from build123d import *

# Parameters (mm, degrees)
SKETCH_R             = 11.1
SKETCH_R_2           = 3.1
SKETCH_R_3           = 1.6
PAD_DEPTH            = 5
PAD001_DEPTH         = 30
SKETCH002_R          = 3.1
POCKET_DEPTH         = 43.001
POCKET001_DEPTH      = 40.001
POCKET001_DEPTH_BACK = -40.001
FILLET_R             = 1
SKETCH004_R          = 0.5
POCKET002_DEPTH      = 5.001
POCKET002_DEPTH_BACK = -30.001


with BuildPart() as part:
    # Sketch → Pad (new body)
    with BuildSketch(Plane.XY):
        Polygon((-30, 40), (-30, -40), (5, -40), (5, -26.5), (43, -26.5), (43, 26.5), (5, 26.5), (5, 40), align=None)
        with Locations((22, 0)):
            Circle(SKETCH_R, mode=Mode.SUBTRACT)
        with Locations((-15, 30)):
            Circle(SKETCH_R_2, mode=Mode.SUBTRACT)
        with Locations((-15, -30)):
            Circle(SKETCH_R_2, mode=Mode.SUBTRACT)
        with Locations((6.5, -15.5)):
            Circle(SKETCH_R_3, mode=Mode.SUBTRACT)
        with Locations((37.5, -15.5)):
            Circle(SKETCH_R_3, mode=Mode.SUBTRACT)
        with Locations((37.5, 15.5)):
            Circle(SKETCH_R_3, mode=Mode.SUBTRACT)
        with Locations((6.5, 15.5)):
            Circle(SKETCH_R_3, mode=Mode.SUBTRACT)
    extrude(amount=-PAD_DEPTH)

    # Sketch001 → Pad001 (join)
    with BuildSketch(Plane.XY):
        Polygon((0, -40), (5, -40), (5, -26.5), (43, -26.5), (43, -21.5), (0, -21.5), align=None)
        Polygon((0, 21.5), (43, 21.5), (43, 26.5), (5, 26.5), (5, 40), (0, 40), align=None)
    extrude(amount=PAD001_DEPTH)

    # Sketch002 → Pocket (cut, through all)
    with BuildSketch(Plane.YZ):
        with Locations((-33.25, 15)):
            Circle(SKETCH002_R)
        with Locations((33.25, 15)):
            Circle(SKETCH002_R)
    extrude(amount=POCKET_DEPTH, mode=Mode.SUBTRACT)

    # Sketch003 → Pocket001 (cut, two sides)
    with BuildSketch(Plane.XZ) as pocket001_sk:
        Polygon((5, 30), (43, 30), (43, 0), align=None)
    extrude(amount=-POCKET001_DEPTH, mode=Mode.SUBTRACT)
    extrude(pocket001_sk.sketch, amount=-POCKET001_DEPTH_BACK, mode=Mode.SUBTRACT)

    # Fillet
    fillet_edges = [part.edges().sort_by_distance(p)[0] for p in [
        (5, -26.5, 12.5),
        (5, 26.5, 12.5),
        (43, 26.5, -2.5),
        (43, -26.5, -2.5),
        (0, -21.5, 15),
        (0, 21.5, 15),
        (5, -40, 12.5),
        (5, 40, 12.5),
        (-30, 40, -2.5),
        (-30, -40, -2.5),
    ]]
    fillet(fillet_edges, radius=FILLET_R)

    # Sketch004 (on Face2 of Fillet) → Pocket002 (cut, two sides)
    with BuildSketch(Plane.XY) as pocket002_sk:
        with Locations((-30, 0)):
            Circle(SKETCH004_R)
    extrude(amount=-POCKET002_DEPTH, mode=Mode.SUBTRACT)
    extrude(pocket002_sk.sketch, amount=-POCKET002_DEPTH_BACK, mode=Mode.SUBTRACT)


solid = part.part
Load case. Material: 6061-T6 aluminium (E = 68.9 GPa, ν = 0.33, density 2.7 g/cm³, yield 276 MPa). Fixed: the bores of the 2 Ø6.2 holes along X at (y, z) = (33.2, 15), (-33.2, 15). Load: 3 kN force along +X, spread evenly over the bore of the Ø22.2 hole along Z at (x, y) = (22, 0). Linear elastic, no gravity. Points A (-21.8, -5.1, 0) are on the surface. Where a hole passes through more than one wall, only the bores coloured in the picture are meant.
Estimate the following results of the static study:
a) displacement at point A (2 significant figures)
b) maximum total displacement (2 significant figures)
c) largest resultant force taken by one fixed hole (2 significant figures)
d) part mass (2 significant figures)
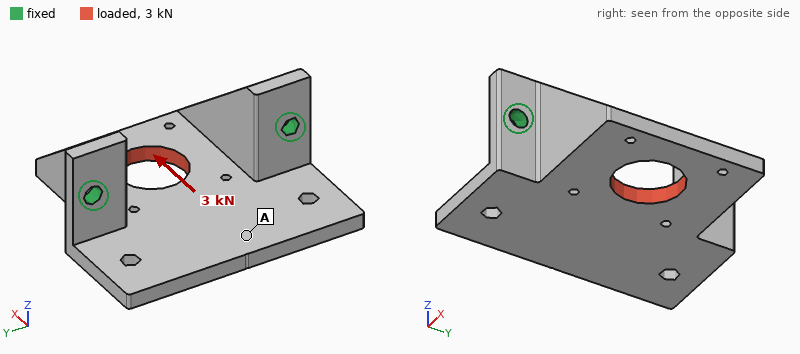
0.16 mm
0.24 mm
1.5 kN
88 g
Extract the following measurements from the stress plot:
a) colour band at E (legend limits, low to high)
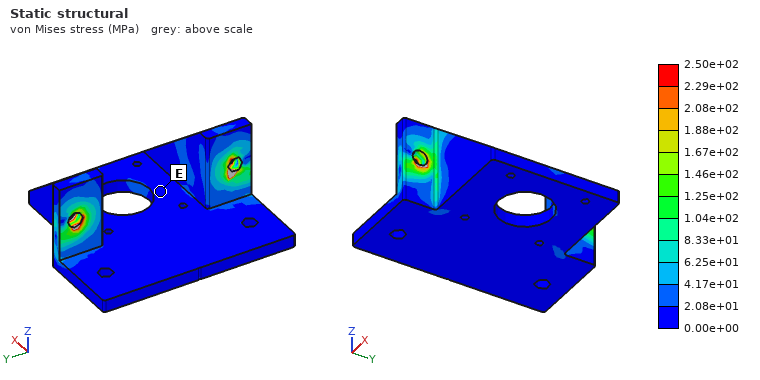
0.00e+00 to 2.08e+01 MPa
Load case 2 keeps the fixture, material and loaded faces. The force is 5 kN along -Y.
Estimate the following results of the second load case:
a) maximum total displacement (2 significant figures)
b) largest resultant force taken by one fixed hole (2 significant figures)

0.19 mm
2.9 kN
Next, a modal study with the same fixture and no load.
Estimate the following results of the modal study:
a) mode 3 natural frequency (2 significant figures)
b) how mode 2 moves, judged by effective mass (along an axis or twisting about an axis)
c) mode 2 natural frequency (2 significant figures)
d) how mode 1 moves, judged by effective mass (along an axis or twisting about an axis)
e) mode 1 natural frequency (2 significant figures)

3800 Hz
twisting about Z
3400 Hz
along X
2000 Hz
